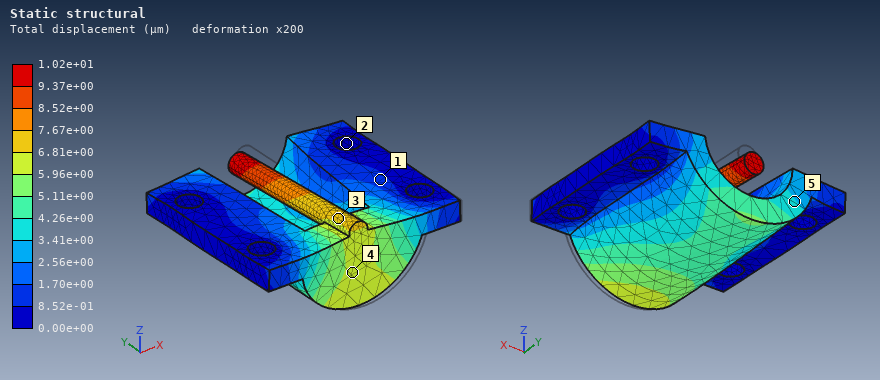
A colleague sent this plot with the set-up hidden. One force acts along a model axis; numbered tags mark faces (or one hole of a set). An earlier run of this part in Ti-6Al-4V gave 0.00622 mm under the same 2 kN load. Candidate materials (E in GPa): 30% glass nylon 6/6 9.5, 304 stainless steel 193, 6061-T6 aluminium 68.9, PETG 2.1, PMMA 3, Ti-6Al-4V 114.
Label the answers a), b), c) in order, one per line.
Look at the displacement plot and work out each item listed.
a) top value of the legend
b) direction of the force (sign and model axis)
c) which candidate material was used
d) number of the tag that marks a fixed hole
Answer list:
a) 1.02e+01 µm
b) +Y
c) 6061-T6 aluminium
d) 2
